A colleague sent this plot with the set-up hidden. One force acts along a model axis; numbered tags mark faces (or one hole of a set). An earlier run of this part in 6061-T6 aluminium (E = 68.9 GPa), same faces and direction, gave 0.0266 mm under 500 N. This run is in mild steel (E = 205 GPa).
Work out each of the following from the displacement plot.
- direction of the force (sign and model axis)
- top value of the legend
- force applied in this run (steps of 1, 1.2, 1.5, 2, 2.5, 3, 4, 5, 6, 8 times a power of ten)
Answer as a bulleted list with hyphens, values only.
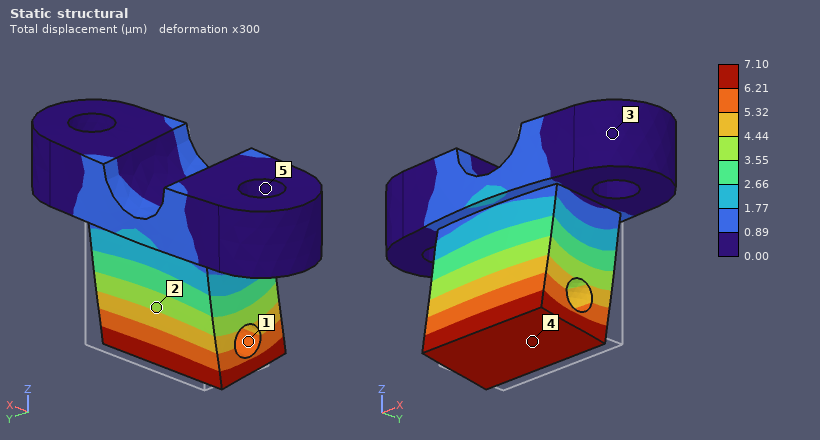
- -Y
- 7.10 µm
- 400 N
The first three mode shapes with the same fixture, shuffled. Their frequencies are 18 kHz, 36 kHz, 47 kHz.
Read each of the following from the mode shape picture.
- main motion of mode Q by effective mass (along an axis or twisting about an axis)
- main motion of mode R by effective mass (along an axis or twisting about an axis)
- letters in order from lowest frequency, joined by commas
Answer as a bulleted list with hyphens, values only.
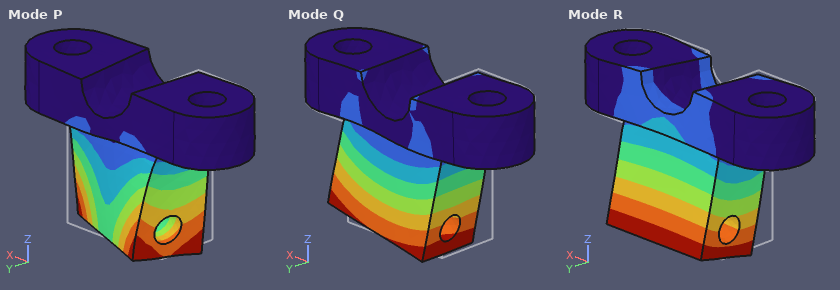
- along X
- along Y
- R, Q, P
